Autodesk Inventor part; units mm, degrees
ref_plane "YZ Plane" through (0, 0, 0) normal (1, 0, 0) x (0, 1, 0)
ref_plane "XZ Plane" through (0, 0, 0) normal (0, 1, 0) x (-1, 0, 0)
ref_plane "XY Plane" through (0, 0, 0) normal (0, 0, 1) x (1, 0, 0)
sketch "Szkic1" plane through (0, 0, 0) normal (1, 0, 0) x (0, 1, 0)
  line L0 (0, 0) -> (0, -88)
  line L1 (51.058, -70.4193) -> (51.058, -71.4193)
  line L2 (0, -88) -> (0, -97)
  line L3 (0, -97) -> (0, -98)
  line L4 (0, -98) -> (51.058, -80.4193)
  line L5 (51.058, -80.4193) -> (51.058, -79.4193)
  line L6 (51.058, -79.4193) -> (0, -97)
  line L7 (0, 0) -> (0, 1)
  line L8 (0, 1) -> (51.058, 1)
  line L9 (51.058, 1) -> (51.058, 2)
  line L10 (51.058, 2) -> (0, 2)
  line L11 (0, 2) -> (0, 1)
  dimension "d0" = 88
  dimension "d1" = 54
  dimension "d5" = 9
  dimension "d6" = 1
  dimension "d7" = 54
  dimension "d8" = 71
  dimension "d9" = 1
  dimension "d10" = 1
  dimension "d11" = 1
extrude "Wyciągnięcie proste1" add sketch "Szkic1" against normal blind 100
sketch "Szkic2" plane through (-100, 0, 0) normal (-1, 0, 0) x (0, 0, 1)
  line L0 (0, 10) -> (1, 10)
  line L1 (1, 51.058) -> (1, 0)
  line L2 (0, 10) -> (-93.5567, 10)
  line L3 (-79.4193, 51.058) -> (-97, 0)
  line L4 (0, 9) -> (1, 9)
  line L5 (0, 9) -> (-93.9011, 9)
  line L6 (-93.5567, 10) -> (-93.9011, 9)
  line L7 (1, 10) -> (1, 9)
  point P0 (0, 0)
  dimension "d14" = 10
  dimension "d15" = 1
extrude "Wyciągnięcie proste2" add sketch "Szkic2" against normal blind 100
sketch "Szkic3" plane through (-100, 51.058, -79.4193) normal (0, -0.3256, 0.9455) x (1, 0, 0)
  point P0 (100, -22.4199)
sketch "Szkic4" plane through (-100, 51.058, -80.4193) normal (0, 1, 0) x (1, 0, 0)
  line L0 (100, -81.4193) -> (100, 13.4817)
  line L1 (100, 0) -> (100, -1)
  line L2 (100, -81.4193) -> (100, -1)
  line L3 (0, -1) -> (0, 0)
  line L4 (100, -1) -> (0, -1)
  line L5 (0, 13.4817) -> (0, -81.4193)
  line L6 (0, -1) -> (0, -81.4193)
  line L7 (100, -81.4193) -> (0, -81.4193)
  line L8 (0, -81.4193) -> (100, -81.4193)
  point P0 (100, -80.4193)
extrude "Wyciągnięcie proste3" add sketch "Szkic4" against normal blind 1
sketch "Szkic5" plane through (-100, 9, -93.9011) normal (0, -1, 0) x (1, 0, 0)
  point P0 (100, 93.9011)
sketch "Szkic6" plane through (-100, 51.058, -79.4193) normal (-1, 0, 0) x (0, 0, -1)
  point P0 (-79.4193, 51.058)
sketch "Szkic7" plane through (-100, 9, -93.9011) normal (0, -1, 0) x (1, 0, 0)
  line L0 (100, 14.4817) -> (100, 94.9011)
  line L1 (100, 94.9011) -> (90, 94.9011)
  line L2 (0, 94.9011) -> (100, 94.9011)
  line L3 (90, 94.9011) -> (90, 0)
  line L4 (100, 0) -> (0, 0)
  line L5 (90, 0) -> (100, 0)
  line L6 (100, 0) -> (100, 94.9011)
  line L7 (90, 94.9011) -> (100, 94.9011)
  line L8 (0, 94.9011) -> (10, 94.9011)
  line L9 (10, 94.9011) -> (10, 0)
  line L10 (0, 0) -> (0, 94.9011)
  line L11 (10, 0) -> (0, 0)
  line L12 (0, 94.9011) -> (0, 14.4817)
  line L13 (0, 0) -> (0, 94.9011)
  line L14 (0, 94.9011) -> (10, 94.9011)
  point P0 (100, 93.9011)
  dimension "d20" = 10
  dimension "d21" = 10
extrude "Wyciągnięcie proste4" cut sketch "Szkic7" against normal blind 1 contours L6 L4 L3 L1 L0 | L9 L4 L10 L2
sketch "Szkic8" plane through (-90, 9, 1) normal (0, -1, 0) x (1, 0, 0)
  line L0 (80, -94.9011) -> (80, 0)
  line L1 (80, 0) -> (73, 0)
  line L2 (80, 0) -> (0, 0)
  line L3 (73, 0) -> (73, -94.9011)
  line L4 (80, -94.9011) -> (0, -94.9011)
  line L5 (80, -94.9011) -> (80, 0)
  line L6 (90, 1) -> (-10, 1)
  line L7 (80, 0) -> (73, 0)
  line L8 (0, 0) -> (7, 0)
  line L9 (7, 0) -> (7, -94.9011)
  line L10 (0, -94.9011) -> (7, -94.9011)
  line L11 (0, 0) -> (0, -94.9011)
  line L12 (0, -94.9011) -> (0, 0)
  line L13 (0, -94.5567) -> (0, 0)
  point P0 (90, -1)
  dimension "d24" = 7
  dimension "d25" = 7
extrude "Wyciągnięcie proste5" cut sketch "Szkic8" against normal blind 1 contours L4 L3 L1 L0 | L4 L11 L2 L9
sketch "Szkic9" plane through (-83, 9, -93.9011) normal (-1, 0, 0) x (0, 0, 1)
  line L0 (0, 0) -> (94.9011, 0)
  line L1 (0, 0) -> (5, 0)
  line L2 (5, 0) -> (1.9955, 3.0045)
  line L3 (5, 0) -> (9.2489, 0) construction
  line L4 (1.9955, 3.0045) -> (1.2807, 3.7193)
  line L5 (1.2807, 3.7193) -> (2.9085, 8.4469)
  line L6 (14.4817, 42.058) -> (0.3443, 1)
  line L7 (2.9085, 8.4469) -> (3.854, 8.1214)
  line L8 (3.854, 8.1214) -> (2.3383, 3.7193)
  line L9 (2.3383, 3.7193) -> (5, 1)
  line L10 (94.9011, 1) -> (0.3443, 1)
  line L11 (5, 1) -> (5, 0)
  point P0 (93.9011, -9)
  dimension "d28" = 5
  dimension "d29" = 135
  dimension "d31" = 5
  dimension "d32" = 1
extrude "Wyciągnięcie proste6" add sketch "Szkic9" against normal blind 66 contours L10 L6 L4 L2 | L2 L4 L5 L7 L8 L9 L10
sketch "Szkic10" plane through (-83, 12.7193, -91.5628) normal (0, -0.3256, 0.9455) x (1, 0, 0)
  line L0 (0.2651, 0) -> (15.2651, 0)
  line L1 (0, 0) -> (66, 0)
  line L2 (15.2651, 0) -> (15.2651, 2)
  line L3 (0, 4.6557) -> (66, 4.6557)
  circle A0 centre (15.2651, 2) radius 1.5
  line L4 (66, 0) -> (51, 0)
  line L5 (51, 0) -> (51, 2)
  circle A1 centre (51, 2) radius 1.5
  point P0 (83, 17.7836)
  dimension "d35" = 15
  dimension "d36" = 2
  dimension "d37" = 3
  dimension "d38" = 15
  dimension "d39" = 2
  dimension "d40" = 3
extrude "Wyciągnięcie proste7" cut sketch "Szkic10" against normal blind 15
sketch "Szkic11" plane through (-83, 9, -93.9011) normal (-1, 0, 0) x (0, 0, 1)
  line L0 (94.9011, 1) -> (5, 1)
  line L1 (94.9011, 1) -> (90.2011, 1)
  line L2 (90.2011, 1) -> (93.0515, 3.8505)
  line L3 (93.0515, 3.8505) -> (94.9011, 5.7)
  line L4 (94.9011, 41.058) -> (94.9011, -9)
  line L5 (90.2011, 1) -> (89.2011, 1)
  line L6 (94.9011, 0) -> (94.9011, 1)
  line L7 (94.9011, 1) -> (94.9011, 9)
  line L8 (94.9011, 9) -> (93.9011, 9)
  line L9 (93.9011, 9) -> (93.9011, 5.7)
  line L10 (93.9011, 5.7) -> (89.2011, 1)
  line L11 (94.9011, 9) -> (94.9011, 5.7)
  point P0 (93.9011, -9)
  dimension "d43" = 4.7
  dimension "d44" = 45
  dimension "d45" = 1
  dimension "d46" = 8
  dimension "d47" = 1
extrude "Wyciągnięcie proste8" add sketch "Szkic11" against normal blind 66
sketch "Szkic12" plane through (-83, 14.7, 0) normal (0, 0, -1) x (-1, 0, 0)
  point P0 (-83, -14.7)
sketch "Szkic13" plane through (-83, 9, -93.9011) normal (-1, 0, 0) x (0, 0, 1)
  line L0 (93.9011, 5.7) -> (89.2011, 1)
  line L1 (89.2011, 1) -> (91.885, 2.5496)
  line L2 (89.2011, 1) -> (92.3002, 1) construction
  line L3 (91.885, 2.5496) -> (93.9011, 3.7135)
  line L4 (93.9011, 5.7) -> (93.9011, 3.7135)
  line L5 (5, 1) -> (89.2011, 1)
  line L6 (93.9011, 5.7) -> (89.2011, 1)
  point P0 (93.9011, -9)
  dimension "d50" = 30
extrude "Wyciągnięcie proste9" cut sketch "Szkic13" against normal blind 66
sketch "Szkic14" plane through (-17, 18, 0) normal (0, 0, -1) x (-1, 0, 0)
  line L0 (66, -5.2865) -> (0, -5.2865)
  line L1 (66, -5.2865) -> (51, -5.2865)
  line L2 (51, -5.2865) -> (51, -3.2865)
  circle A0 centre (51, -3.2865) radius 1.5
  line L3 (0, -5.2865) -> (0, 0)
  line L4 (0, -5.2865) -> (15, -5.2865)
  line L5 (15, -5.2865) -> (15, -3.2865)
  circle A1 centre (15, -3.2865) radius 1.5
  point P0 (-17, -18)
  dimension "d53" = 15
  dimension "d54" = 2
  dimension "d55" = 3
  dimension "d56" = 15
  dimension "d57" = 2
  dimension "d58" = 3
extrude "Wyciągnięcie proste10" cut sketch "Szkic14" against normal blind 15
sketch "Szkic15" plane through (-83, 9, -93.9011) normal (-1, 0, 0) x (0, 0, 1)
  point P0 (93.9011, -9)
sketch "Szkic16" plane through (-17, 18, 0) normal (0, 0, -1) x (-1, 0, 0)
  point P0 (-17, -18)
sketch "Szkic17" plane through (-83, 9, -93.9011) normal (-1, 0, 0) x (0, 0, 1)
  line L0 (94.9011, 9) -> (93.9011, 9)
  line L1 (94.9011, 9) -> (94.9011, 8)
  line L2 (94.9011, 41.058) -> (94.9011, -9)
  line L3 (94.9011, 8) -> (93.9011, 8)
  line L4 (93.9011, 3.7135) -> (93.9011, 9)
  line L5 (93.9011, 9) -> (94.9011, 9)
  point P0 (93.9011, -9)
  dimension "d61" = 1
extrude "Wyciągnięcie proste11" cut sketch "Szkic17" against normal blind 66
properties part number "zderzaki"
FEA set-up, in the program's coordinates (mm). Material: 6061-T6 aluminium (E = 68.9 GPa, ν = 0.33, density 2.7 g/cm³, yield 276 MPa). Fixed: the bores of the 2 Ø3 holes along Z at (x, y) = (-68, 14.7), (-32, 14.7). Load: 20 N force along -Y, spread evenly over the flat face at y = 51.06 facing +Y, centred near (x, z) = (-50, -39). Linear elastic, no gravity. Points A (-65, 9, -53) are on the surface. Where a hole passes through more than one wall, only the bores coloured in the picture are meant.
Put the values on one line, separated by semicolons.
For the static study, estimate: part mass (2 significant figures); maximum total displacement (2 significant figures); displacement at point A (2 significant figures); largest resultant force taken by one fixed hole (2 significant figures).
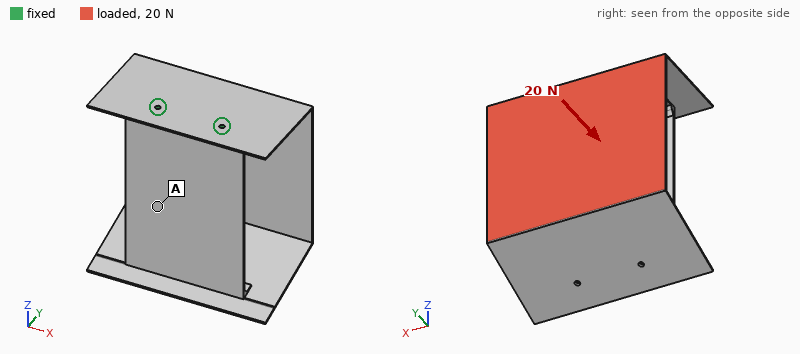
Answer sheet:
71 g; 1.7 mm; 0.80 mm; 10 N
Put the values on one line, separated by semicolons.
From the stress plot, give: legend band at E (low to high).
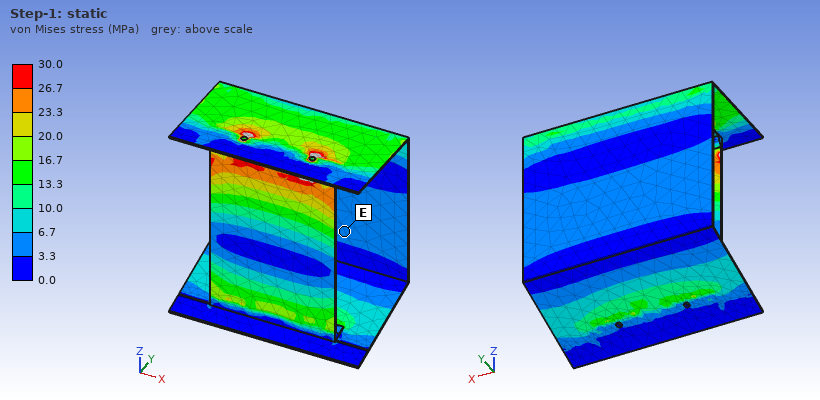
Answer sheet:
3.3 to 6.7 MPa
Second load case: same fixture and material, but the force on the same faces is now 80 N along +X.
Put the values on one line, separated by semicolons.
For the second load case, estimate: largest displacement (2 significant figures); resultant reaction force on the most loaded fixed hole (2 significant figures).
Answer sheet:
1.7 mm; 120 N
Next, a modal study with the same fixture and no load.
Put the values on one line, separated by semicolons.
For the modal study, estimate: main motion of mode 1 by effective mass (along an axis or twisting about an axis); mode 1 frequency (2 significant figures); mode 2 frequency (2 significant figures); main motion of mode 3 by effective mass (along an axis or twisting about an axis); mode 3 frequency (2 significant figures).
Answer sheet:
along Y; 71 Hz; 200 Hz; along Z; 270 Hz
